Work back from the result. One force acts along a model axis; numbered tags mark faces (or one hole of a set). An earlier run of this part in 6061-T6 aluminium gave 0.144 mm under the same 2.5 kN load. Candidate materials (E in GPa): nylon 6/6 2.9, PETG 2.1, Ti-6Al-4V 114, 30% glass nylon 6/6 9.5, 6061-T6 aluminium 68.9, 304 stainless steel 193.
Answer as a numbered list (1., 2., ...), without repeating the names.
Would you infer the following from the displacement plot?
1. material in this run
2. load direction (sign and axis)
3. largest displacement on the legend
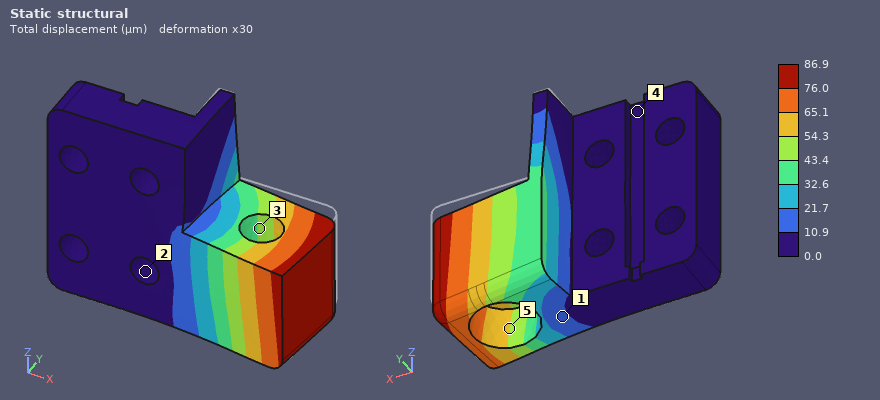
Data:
1. Ti-6Al-4V
2. -Y
3. 86.9 µm
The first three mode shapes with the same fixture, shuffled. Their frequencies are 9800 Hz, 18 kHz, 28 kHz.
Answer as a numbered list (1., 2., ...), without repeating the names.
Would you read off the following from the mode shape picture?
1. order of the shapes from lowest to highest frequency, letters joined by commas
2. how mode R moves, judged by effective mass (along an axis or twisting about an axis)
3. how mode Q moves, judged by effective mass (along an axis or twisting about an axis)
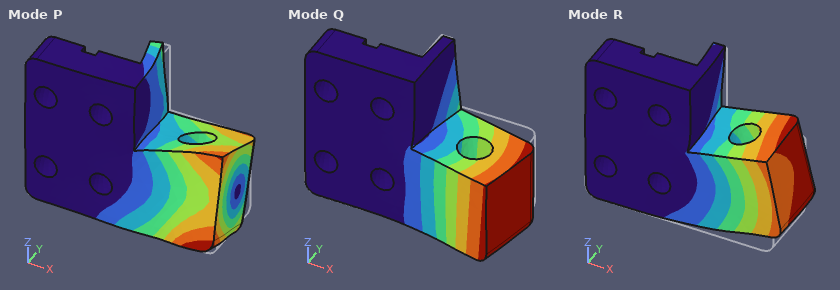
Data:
1. Q, R, P
2. along Z
3. along Y
